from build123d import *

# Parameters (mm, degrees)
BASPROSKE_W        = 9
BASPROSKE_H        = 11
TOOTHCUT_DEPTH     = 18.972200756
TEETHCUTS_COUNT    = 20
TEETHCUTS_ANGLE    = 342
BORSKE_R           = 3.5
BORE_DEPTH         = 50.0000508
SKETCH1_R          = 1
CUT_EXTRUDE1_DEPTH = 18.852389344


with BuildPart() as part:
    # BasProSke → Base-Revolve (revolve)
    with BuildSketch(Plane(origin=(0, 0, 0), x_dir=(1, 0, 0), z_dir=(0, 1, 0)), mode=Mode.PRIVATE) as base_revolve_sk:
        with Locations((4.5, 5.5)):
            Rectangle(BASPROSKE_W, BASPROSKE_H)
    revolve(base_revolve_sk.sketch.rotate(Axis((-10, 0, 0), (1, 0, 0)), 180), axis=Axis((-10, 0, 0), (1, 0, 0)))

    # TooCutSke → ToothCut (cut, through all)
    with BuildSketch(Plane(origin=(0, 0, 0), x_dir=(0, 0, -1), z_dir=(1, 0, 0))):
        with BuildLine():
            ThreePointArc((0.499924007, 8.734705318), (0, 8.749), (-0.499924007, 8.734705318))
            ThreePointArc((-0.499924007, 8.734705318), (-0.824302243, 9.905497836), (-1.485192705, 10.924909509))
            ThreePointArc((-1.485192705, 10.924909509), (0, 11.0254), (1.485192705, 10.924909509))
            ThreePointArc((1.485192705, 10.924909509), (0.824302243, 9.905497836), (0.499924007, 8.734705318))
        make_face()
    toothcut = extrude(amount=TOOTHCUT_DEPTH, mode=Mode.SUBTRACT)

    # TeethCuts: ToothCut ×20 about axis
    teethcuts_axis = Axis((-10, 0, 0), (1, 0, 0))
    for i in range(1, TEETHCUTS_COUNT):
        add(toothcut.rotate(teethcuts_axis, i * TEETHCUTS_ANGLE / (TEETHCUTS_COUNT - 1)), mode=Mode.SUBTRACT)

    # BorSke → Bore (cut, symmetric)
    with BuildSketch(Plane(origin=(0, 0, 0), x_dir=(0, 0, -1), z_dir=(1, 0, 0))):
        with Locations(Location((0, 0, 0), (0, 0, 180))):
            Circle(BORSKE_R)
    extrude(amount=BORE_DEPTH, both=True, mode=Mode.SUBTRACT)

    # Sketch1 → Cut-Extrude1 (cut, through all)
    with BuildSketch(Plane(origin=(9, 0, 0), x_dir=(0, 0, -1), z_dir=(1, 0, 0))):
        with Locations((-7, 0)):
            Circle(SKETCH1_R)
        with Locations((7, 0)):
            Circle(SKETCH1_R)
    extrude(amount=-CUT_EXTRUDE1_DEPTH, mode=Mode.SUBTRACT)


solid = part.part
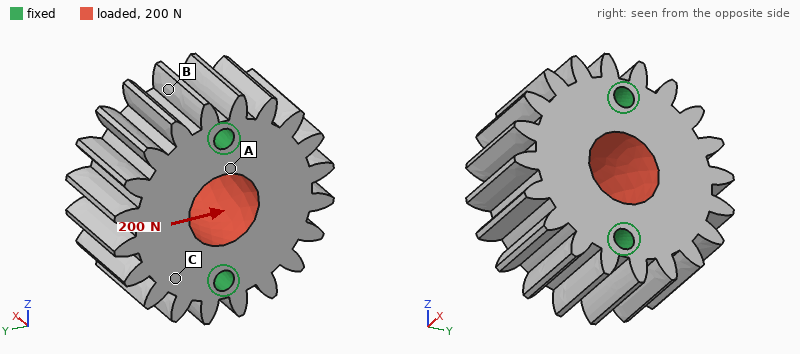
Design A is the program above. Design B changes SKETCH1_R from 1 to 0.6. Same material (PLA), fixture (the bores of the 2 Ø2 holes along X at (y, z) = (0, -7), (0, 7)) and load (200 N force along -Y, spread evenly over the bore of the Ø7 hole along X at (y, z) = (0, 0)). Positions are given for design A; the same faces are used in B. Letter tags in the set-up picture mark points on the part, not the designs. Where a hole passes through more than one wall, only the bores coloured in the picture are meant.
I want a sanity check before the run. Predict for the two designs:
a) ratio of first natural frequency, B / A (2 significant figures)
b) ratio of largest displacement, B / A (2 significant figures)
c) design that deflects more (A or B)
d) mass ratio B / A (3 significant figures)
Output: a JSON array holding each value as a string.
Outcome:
["0.88", "1.1", "B", "1.02"]
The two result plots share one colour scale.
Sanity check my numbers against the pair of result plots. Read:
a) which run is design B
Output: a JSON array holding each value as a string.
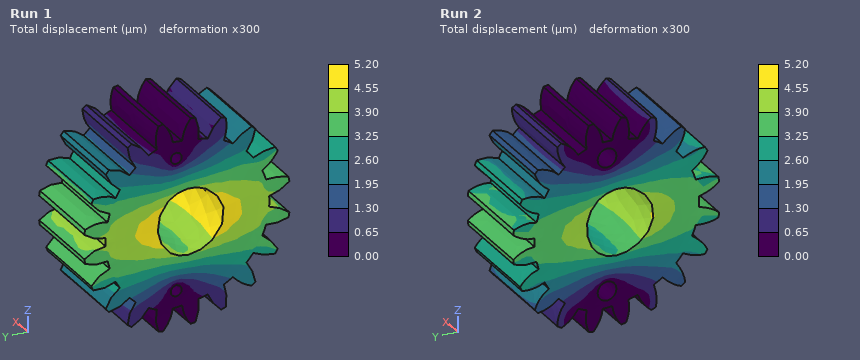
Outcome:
["Run 1"]
